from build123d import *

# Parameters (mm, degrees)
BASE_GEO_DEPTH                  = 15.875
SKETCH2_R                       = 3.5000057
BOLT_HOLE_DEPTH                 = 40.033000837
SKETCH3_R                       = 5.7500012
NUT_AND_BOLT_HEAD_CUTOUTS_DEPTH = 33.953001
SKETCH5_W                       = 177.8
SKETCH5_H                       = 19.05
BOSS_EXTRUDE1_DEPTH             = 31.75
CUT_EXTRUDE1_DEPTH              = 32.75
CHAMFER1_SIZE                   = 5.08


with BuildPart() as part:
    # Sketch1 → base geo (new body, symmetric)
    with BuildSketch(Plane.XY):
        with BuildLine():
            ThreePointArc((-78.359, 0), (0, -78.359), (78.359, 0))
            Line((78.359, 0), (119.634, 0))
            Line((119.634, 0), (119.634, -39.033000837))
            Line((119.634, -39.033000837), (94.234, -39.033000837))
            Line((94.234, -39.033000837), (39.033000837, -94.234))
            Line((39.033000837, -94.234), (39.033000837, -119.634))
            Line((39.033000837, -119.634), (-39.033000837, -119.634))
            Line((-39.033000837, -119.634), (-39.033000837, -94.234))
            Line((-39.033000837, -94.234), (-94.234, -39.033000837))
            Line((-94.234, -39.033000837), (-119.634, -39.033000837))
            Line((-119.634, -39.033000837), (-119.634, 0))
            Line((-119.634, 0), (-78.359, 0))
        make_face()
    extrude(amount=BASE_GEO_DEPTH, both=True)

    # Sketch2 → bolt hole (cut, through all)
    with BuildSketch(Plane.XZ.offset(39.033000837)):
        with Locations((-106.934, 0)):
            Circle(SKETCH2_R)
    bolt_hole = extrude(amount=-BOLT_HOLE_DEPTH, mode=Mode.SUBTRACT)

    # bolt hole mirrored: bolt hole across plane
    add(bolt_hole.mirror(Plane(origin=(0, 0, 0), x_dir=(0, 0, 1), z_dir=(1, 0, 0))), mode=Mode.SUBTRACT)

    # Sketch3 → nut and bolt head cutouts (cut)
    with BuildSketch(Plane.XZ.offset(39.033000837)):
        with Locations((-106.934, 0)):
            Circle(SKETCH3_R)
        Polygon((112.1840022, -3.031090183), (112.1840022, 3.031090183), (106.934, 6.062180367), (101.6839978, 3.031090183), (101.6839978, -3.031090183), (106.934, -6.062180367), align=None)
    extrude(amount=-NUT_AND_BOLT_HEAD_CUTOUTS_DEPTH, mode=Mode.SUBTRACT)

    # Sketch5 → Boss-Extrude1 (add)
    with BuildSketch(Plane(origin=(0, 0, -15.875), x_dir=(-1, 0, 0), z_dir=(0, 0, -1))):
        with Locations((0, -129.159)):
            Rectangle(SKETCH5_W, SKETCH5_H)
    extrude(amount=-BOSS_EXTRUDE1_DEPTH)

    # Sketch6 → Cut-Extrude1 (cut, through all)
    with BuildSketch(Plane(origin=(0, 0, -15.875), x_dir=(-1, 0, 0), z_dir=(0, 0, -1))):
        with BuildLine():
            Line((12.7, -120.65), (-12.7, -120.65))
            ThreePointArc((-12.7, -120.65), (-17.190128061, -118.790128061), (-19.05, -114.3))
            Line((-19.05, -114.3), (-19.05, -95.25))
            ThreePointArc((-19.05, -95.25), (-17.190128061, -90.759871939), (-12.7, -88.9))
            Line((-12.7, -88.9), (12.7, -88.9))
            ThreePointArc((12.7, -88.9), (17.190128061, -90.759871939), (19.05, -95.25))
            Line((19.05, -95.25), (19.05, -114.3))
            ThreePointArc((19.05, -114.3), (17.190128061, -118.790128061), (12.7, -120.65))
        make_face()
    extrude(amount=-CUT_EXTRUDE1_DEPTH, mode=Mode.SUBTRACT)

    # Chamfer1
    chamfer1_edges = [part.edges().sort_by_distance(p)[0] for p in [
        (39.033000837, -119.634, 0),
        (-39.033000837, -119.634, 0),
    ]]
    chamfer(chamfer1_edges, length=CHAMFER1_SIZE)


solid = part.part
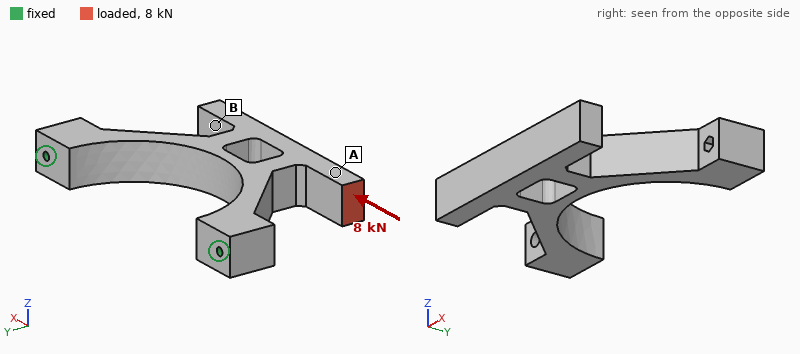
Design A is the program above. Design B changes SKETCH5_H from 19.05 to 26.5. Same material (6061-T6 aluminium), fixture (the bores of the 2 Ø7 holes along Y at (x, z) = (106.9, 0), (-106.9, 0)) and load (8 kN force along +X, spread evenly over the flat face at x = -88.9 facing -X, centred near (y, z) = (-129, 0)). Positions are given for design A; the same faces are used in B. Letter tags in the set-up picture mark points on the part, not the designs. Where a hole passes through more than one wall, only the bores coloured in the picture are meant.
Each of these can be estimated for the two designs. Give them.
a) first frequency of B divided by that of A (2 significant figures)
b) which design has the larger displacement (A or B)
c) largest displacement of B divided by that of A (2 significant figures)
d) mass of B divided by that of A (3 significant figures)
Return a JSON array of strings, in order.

["0.91", "A", "0.89", "1.09"]
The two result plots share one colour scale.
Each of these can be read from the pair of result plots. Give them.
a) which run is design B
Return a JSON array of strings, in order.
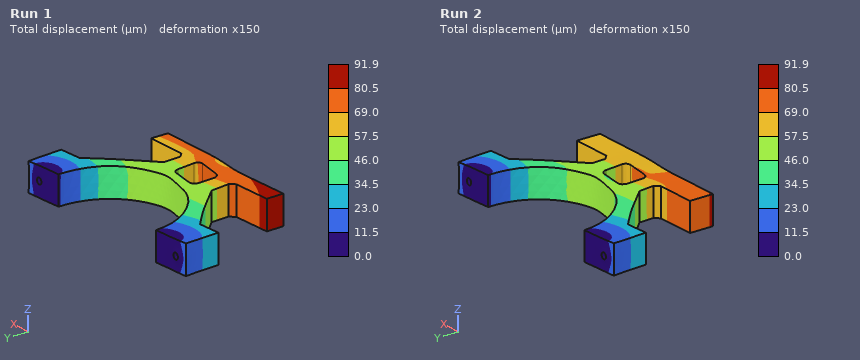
["Run 2"]
